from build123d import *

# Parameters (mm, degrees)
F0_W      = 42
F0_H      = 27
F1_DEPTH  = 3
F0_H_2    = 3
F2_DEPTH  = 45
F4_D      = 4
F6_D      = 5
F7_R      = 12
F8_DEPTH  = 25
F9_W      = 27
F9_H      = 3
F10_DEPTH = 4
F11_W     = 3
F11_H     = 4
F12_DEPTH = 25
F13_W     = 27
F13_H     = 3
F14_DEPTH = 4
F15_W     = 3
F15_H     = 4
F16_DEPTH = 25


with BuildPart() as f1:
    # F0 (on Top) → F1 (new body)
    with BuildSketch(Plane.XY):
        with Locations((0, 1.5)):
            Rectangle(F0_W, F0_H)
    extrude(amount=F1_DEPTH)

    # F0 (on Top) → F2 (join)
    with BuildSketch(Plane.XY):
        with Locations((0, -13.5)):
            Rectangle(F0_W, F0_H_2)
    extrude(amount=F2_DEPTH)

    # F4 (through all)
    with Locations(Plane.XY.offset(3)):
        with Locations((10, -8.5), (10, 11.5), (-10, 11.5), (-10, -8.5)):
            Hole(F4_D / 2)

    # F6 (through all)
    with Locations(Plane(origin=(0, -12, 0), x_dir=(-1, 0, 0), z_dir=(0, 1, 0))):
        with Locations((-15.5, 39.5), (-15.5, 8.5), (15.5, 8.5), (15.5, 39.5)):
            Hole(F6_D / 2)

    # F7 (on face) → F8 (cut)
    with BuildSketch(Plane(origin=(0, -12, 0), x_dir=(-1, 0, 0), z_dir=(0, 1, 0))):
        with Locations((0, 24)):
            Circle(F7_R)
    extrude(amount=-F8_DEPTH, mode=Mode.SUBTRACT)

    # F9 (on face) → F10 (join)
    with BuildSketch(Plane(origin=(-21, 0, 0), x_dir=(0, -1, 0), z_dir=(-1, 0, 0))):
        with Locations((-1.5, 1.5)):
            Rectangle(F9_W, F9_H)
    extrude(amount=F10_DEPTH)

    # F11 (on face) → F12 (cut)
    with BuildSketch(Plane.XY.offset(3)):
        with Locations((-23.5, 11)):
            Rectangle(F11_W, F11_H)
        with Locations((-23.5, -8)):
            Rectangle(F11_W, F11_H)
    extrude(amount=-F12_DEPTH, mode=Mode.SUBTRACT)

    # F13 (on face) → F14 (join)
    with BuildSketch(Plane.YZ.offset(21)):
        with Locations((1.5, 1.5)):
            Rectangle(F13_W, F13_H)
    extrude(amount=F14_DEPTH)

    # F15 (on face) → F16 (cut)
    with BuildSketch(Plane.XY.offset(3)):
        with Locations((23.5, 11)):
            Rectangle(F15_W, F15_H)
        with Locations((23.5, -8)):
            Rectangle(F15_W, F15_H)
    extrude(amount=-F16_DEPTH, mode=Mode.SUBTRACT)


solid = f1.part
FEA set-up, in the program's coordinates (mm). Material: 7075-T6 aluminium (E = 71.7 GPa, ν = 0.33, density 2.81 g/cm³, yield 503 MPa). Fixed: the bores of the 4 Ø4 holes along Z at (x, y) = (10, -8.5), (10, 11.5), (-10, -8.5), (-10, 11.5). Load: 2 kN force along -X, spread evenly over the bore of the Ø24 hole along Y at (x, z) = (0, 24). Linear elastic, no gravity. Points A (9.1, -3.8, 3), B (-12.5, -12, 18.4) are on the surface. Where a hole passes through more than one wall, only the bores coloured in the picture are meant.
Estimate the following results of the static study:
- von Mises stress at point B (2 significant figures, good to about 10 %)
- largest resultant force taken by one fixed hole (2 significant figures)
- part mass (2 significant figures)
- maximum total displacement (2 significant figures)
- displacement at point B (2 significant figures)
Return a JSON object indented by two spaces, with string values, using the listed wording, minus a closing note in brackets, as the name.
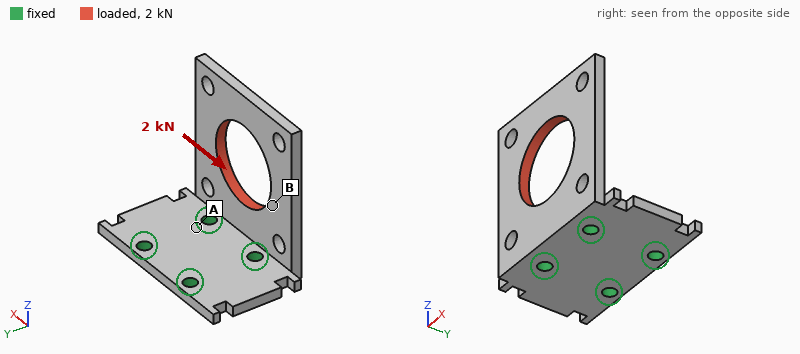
{
  "von Mises stress at point B": "53 MPa",
  "largest resultant force taken by one fixed hole": "2.2 kN",
  "part mass": "22 g",
  "maximum total displacement": "0.26 mm",
  "displacement at point B": "0.10 mm"
}
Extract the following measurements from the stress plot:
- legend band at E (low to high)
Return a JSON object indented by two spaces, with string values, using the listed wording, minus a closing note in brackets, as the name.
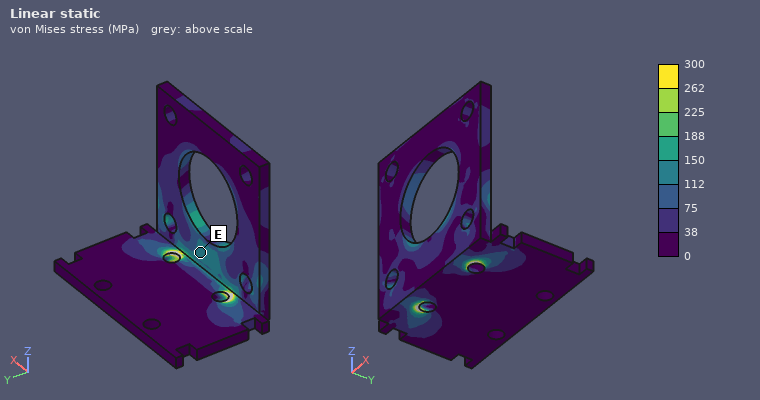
{
  "legend band at E": "112 to 150 MPa"
}
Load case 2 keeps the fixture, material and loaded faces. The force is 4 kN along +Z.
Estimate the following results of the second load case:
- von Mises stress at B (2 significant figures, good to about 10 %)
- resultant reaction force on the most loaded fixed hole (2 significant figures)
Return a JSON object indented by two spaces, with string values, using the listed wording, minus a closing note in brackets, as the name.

{
  "von Mises stress at B": "73 MPa",
  "resultant reaction force on the most loaded fixed hole": "2.1 kN"
}
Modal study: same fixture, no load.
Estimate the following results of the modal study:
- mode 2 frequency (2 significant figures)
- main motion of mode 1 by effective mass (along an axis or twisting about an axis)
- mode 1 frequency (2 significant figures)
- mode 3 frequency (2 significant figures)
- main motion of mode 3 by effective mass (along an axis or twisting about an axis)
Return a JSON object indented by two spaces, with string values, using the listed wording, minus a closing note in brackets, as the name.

{
  "mode 2 frequency": "2500 Hz",
  "main motion of mode 1 by effective mass": "along Y",
  "mode 1 frequency": "1100 Hz",
  "mode 3 frequency": "5100 Hz",
  "main motion of mode 3 by effective mass": "along X"
}
